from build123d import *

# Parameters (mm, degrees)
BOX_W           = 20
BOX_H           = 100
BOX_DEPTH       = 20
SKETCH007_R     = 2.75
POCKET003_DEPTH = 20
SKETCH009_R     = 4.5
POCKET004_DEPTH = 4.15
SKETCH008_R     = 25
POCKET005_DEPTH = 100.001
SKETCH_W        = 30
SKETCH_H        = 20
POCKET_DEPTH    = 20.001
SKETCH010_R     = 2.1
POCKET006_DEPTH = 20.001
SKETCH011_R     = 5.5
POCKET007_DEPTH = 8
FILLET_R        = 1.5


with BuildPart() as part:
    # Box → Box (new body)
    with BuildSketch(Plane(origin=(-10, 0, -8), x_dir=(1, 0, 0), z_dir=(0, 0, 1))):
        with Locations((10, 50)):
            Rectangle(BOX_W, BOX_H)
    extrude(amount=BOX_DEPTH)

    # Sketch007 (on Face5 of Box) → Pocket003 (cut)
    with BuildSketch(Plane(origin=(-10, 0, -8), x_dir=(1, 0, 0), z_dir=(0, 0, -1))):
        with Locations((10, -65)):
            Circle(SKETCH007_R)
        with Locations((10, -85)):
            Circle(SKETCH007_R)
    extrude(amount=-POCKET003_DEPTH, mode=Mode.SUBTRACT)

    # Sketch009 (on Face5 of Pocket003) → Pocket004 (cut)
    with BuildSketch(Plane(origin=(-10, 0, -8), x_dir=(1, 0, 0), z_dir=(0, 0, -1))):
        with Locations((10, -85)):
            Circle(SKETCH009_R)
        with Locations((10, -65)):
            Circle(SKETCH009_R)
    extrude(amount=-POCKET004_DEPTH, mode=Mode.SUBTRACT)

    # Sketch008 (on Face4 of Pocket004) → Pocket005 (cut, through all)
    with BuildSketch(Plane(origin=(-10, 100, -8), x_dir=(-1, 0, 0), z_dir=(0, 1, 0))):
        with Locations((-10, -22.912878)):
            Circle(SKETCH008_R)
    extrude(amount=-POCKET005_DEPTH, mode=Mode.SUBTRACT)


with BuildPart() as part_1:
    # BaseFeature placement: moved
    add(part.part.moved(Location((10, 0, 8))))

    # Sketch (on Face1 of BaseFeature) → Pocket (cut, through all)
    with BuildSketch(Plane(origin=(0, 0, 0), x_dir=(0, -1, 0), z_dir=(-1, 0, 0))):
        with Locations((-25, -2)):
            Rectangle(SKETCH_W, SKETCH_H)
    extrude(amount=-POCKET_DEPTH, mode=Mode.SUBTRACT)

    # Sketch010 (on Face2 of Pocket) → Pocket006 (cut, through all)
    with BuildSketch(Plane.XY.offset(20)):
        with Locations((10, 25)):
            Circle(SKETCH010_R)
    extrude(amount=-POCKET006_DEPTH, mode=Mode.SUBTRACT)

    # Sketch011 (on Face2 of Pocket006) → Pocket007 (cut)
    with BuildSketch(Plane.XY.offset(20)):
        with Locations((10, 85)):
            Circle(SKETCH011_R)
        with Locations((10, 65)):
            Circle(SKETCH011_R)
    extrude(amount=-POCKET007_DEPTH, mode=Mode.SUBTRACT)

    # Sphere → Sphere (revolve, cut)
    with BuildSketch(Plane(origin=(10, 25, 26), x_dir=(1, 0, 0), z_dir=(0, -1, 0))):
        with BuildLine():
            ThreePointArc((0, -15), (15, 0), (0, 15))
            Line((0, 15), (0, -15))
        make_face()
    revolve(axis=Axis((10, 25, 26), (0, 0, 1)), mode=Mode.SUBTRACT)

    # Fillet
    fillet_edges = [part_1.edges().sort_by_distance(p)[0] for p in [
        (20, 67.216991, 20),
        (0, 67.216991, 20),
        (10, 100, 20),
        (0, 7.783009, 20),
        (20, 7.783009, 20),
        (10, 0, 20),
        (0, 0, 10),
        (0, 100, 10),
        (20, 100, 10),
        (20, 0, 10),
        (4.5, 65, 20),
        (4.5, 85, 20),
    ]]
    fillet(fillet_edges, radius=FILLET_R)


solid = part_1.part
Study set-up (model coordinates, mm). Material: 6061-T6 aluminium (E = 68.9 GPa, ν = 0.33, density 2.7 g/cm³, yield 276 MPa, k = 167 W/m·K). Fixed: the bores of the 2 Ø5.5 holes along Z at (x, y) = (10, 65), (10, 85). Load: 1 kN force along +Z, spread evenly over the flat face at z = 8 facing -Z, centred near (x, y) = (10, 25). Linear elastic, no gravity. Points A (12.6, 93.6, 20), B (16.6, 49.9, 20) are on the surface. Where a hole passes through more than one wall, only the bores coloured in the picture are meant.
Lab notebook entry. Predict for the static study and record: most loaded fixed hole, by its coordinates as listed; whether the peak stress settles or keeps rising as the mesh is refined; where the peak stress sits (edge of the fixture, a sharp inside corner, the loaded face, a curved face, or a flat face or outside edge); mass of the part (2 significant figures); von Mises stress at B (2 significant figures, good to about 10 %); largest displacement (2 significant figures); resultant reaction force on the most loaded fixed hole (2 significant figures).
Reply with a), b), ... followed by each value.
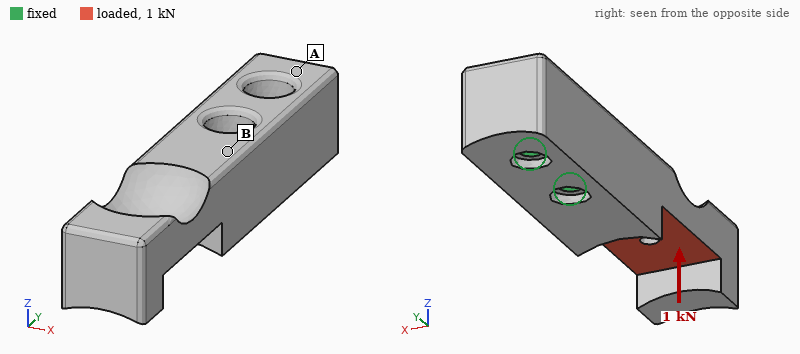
a) (10, 65)
b) keeps rising
c) edge of the fixture
d) 76 g
e) 26 MPa
f) 0.28 mm
g) 2.3 kN
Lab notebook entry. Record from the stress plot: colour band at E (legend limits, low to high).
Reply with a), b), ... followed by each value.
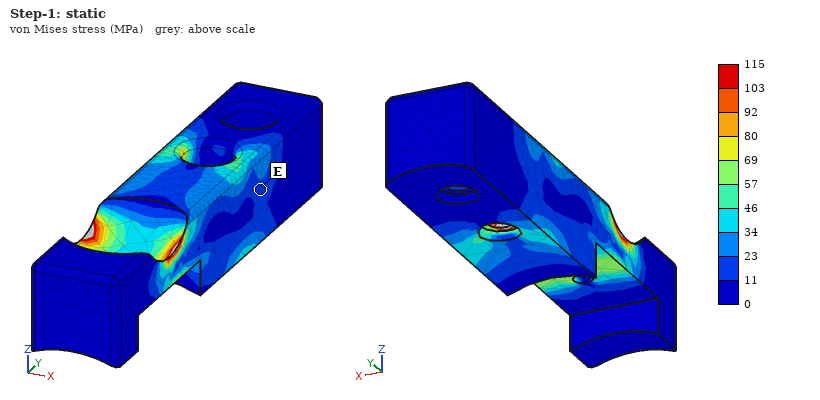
a) 11 to 23 MPa
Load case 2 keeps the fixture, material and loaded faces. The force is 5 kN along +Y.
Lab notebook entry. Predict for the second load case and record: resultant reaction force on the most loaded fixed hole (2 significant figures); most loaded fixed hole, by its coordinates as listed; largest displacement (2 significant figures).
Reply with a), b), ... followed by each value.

a) 4.0 kN
b) (10, 65)
c) 0.30 mm
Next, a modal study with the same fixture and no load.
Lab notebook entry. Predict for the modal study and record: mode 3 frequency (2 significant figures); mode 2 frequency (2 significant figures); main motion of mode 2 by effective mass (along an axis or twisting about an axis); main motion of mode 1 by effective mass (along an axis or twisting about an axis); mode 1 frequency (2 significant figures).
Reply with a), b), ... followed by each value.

a) 5900 Hz
b) 3000 Hz
c) along X
d) along Z
e) 1700 Hz
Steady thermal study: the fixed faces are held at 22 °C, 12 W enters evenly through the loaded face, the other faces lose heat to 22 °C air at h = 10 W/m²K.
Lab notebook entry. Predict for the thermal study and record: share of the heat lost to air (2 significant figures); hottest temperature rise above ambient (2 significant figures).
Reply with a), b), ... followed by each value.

a) 3.6 %
b) 15 K
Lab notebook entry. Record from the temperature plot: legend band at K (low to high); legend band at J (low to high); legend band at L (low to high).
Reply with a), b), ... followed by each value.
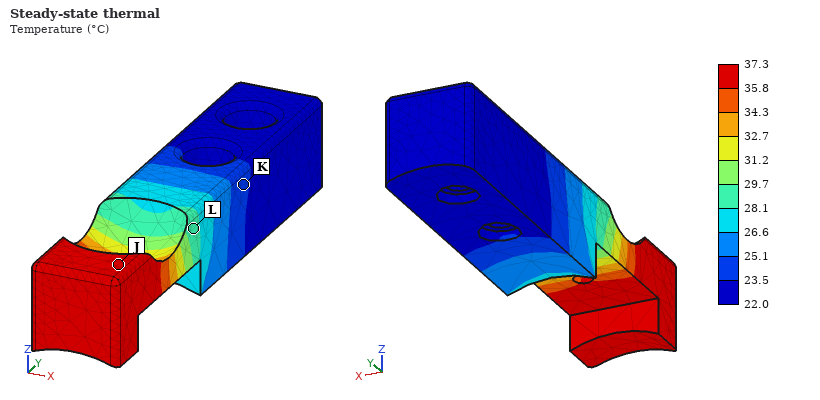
a) 23.5 to 25.1 °C
b) 35.8 to 37.3 °C
c) 28.1 to 29.7 °C
